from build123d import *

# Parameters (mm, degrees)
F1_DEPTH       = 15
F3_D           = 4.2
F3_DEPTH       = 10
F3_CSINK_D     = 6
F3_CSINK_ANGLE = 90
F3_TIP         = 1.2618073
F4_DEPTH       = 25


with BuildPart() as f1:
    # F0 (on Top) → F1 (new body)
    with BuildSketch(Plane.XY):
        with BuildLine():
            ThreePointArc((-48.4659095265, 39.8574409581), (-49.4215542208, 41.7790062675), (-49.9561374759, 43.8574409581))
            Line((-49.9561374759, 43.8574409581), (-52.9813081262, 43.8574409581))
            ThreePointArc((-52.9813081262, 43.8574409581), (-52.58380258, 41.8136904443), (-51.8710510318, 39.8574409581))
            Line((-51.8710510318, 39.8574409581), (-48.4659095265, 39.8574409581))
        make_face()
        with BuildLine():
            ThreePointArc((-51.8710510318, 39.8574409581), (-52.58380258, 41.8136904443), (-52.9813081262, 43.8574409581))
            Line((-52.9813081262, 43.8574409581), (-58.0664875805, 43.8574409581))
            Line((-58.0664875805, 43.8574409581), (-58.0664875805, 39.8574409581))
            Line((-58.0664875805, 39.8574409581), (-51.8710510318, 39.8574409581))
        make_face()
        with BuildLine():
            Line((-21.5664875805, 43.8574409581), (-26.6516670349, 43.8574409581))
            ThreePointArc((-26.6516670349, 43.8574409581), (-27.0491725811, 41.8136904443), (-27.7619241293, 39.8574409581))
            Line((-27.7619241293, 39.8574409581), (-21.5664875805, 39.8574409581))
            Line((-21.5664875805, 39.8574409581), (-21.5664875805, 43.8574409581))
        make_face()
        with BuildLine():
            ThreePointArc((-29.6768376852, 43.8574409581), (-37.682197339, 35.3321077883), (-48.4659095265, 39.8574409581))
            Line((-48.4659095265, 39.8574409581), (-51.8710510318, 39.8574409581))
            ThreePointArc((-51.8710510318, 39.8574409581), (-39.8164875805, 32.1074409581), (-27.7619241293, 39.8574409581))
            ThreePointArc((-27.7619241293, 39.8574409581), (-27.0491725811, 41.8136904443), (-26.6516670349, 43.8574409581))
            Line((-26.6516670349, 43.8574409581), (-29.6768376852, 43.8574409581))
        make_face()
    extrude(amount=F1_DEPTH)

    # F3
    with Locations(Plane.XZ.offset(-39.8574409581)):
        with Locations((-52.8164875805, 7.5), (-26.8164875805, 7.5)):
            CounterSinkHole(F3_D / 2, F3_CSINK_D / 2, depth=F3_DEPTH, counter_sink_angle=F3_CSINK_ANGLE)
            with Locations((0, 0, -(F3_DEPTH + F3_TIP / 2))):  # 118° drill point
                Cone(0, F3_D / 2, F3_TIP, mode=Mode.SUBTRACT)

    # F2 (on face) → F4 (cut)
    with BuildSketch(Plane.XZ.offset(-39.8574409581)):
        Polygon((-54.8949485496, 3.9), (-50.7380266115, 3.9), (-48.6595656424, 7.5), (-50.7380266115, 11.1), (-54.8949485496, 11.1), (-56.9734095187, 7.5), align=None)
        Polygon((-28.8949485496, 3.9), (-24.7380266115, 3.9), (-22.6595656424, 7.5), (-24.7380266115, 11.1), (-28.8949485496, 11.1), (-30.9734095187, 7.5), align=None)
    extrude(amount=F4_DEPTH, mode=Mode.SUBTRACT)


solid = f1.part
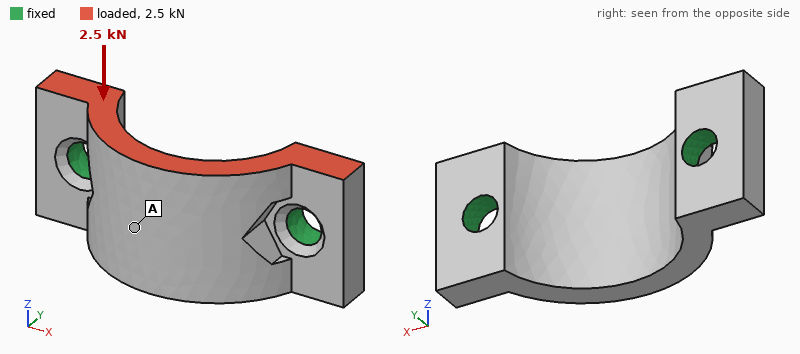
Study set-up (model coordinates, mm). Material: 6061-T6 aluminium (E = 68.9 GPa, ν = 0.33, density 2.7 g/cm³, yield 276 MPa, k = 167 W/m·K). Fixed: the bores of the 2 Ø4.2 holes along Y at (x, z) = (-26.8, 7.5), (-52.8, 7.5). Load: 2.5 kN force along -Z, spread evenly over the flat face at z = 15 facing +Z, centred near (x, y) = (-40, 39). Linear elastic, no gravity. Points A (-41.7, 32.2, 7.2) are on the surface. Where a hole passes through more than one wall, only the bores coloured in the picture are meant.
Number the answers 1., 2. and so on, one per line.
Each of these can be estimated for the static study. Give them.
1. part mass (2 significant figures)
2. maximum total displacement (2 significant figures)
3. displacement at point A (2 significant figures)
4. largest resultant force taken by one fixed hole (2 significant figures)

1. 5.4 g
2. 40 µm
3. 31 µm
4. 1.3 kN
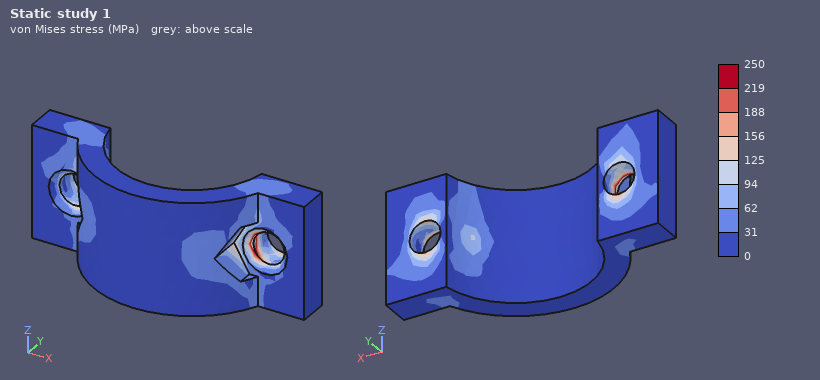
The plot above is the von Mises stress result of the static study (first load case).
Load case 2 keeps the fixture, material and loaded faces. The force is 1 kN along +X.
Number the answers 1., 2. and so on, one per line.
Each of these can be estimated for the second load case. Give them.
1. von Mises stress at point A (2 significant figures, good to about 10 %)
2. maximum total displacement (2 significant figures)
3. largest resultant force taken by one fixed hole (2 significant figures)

1. 8.7 MPa
2. 15 µm
3. 530 N
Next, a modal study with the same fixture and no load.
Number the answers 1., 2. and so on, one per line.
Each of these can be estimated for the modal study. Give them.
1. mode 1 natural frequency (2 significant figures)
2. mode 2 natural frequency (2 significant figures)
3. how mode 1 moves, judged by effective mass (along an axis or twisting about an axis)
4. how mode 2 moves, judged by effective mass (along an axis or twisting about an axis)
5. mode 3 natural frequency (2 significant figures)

1. 19 kHz
2. 29 kHz
3. along Z
4. along X
5. 35 kHz
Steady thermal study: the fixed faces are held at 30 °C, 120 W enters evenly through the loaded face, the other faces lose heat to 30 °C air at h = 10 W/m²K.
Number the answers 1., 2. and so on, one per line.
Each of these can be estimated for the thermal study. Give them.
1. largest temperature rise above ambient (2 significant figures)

1. 79 K
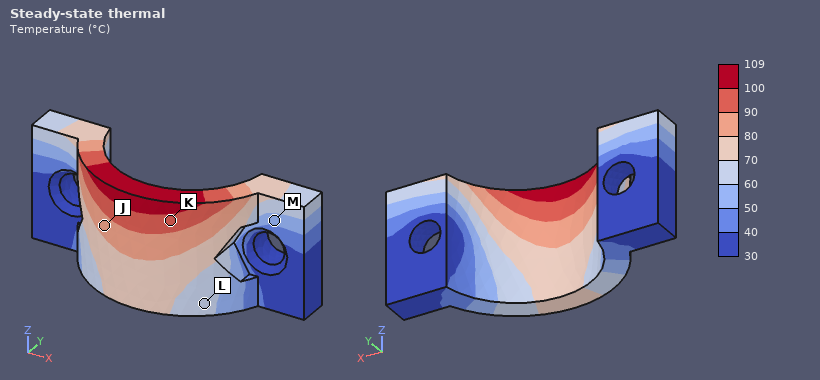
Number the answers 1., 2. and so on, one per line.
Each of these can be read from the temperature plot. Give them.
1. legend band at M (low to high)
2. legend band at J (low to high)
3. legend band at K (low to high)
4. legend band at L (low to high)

1. 50 to 60 °C
2. 80 to 90 °C
3. 90 to 100 °C
4. 60 to 70 °C
